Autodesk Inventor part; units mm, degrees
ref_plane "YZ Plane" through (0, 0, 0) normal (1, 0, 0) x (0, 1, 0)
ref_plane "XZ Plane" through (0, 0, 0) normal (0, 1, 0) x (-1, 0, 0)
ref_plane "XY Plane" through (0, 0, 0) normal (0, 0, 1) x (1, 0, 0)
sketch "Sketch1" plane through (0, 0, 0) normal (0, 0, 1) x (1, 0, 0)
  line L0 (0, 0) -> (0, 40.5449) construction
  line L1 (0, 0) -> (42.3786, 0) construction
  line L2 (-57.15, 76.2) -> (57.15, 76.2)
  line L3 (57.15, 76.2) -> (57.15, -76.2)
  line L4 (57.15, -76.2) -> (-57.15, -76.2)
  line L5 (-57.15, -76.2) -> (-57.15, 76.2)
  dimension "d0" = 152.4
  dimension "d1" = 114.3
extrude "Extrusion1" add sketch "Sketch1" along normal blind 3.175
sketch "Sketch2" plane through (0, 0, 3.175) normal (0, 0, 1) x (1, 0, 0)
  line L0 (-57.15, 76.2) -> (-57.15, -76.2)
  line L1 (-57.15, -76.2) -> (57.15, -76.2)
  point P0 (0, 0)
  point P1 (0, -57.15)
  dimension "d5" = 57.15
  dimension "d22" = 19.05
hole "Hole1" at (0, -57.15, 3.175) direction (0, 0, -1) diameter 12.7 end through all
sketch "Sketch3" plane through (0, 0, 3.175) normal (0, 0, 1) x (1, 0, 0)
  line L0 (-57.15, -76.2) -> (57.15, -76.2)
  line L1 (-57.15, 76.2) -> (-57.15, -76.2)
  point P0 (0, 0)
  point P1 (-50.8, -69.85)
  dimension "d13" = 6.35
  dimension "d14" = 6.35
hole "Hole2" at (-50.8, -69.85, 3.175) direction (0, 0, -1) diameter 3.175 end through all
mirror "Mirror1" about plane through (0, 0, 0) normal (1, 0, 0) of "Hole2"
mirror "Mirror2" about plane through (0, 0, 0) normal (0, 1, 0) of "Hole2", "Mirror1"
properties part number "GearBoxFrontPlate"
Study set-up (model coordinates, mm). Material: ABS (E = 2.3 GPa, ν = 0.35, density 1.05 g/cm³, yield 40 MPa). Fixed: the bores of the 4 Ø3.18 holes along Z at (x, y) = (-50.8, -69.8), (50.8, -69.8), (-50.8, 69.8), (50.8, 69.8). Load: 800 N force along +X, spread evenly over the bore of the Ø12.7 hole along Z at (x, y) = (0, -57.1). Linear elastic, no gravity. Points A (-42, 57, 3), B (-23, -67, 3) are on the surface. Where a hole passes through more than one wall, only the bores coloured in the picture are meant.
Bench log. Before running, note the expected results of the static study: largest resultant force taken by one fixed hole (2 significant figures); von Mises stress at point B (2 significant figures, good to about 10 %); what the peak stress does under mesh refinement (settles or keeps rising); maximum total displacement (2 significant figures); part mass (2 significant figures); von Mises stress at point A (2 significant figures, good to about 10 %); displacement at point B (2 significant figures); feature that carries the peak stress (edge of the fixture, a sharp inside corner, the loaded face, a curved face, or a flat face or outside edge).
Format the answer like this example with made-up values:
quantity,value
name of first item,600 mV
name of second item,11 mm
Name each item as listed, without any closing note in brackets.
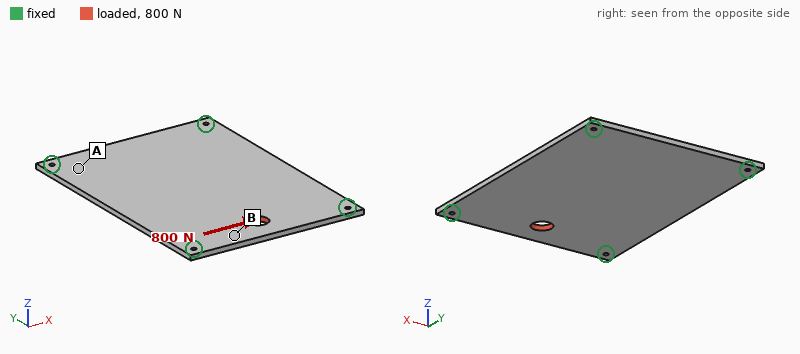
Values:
quantity,value
largest resultant force taken by one fixed hole,350 N
von Mises stress at point B,4.6 MPa
what the peak stress does under mesh refinement,keeps rising
maximum total displacement,0.13 mm
part mass,58 g
von Mises stress at point A,1.2 MPa
displacement at point B,0.080 mm
feature that carries the peak stress,edge of the fixture
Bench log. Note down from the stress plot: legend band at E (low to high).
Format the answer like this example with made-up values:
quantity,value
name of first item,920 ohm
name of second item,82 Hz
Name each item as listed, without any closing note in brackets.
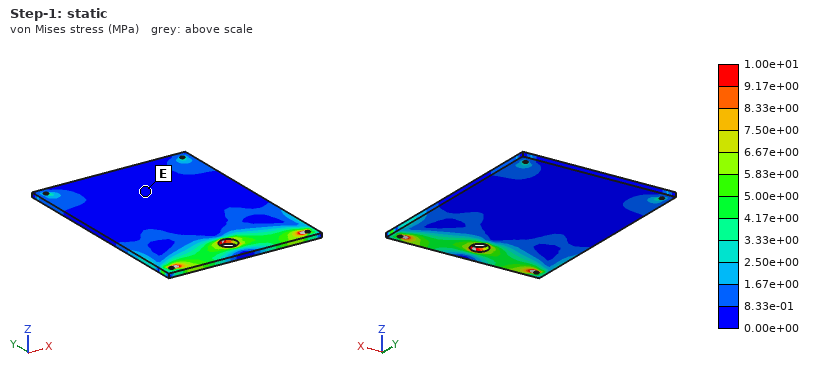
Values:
quantity,value
legend band at E,0.00e+00 to 8.33e-01 MPa
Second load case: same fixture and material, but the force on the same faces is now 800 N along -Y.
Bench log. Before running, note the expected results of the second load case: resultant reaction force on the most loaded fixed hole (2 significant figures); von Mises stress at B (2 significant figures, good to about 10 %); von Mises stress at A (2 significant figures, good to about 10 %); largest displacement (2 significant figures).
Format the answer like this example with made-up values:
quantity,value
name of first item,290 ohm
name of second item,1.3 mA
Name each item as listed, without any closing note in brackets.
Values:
quantity,value
resultant reaction force on the most loaded fixed hole,250 N
von Mises stress at B,1.7 MPa
von Mises stress at A,2.2 MPa
largest displacement,0.21 mm
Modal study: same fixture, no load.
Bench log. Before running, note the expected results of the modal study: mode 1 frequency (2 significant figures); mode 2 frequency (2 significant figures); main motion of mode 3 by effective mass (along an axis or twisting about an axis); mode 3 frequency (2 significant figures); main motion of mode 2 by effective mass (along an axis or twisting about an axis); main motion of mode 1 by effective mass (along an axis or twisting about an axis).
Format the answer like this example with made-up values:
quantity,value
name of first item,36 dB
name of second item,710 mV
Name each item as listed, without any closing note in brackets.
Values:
quantity,value
mode 1 frequency,180 Hz
mode 2 frequency,300 Hz
main motion of mode 3 by effective mass,twisting about X
mode 3 frequency,420 Hz
main motion of mode 2 by effective mass,twisting about Y
main motion of mode 1 by effective mass,along Z
